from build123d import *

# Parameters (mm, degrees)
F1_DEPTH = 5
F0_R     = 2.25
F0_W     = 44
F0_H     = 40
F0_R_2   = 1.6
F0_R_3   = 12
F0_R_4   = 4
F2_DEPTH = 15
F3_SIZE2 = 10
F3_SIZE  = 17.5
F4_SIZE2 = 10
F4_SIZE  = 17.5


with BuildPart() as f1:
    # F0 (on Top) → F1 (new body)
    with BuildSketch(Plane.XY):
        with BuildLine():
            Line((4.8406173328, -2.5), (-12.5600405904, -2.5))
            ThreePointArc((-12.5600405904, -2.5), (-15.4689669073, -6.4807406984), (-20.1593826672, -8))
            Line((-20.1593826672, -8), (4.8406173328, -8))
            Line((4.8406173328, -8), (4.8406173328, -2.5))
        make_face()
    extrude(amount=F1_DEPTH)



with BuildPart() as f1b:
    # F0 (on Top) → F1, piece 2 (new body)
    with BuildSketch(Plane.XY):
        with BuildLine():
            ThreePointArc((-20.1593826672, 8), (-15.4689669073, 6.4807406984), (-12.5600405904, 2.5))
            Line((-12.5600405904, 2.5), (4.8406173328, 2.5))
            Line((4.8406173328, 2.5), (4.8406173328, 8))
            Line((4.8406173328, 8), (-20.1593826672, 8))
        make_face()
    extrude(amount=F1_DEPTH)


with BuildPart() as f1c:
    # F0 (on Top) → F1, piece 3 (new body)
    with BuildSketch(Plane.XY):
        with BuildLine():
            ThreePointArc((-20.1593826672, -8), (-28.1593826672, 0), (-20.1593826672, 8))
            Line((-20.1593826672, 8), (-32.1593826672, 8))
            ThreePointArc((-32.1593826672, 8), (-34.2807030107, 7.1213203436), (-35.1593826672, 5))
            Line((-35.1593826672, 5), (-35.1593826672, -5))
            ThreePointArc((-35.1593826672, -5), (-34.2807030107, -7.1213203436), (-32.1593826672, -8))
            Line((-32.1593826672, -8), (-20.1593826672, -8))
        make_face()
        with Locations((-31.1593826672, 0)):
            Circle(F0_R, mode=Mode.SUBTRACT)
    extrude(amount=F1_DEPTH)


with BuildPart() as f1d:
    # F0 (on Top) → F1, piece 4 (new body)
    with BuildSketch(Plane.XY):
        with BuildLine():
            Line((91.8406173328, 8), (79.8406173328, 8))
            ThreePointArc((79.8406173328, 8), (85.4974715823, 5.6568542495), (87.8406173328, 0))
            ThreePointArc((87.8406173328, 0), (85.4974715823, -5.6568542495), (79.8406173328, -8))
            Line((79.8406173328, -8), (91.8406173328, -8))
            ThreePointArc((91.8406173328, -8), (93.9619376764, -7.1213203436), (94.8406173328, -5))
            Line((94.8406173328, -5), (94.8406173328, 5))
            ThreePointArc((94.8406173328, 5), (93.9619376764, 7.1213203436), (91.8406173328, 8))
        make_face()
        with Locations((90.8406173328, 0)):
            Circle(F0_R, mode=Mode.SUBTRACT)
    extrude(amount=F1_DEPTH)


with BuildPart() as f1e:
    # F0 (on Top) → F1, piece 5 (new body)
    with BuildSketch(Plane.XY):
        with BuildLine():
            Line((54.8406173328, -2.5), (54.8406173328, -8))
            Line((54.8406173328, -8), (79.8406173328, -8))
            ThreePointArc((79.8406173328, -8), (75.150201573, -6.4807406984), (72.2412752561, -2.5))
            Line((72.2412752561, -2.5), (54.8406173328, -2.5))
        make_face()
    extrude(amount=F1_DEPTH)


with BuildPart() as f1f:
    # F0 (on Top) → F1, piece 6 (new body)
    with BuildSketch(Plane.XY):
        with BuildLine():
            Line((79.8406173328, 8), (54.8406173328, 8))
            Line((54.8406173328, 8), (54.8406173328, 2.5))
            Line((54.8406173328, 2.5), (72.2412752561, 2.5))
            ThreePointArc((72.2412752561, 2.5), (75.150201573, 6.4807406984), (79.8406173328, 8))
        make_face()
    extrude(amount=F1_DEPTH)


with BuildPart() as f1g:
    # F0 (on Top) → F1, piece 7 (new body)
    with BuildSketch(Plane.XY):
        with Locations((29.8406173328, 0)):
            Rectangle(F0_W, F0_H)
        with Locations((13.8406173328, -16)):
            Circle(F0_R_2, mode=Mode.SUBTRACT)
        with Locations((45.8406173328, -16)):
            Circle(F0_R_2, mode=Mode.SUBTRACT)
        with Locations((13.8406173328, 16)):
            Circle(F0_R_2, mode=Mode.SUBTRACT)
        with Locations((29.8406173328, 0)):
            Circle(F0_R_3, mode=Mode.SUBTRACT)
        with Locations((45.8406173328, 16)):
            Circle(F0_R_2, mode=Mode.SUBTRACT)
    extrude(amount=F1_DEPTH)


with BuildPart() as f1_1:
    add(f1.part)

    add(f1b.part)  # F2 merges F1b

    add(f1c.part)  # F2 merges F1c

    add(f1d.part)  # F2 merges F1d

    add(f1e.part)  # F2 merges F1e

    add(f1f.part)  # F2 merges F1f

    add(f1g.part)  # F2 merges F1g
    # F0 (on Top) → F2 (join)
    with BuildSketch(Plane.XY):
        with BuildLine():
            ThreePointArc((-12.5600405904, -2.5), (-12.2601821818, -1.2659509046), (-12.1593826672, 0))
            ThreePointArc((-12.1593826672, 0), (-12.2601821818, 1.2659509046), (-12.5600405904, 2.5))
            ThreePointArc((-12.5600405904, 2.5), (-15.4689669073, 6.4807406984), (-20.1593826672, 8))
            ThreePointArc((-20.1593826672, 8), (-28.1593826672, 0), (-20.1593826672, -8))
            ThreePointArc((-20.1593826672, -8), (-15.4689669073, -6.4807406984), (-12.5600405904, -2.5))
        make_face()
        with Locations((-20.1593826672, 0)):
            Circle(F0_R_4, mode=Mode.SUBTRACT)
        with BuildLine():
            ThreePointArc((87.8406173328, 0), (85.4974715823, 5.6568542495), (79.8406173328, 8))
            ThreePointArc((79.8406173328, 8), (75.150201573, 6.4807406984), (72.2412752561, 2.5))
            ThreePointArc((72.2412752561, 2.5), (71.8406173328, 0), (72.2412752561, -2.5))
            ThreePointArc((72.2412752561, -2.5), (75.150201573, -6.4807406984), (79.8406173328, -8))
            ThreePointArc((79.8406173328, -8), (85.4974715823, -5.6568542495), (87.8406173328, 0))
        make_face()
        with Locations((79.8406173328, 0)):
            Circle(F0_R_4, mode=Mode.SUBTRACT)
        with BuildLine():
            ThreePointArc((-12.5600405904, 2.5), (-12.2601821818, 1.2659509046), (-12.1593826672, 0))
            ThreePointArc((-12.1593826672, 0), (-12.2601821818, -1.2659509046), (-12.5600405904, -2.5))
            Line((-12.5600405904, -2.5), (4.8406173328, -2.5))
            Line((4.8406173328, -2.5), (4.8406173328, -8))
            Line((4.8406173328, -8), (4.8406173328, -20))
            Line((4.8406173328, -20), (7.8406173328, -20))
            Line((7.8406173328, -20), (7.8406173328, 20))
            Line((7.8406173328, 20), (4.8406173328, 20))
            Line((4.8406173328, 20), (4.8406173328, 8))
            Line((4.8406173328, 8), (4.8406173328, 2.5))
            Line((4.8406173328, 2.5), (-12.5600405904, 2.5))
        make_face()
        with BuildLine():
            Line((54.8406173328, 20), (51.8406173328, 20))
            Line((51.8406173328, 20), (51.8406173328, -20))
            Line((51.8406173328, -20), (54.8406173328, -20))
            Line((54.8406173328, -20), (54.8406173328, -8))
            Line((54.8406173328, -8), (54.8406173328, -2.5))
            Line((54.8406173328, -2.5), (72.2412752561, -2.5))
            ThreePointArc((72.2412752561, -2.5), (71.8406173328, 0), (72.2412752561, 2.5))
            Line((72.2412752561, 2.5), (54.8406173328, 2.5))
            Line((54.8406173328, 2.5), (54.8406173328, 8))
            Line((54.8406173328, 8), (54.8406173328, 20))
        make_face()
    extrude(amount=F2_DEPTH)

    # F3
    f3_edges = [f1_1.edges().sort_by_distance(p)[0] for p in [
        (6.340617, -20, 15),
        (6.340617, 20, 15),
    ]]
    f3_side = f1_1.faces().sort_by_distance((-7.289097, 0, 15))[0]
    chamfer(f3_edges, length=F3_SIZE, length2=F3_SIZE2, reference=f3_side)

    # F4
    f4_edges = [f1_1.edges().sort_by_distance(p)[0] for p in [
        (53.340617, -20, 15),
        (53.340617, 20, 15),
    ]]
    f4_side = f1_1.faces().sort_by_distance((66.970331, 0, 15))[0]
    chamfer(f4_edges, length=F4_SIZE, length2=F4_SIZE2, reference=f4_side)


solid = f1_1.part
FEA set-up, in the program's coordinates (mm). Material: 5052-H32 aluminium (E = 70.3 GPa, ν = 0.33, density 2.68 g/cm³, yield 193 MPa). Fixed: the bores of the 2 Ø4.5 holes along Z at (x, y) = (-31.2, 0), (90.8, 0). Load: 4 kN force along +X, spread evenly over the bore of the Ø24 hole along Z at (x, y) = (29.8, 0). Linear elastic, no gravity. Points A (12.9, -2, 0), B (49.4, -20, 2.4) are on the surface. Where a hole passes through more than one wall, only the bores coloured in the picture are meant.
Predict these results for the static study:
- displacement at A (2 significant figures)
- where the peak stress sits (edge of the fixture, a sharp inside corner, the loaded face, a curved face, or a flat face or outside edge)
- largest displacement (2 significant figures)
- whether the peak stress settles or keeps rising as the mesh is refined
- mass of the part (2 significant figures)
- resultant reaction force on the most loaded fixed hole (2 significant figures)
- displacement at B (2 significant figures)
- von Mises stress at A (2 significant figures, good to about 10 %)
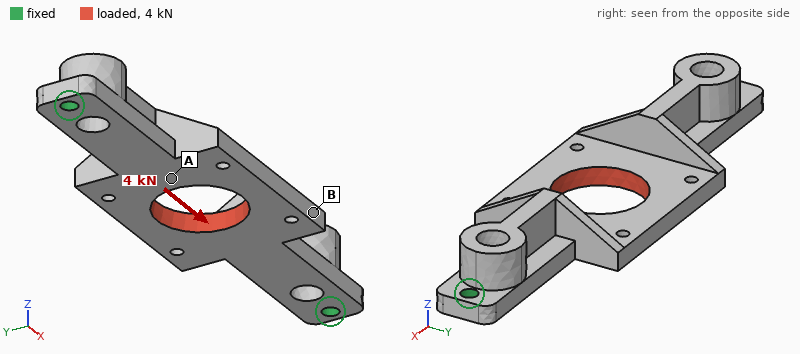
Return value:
18 µm
edge of the fixture
24 µm
keeps rising
52 g
2.0 kN
22 µm
16 MPa
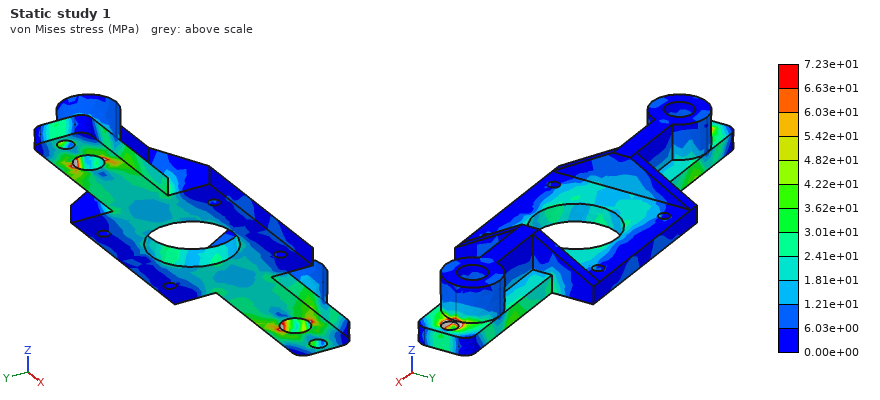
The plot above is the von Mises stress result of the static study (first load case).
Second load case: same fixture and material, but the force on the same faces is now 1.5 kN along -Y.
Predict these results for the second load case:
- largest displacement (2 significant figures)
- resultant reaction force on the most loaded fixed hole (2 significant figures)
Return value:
97 µm
750 N
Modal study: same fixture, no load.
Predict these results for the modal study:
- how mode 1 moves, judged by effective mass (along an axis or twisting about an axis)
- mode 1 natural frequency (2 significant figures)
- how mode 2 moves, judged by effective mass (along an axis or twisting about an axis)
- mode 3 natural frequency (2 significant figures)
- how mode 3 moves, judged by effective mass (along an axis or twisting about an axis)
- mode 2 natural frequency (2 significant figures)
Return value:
along Z
1500 Hz
twisting about X
3700 Hz
along Y
3400 Hz
